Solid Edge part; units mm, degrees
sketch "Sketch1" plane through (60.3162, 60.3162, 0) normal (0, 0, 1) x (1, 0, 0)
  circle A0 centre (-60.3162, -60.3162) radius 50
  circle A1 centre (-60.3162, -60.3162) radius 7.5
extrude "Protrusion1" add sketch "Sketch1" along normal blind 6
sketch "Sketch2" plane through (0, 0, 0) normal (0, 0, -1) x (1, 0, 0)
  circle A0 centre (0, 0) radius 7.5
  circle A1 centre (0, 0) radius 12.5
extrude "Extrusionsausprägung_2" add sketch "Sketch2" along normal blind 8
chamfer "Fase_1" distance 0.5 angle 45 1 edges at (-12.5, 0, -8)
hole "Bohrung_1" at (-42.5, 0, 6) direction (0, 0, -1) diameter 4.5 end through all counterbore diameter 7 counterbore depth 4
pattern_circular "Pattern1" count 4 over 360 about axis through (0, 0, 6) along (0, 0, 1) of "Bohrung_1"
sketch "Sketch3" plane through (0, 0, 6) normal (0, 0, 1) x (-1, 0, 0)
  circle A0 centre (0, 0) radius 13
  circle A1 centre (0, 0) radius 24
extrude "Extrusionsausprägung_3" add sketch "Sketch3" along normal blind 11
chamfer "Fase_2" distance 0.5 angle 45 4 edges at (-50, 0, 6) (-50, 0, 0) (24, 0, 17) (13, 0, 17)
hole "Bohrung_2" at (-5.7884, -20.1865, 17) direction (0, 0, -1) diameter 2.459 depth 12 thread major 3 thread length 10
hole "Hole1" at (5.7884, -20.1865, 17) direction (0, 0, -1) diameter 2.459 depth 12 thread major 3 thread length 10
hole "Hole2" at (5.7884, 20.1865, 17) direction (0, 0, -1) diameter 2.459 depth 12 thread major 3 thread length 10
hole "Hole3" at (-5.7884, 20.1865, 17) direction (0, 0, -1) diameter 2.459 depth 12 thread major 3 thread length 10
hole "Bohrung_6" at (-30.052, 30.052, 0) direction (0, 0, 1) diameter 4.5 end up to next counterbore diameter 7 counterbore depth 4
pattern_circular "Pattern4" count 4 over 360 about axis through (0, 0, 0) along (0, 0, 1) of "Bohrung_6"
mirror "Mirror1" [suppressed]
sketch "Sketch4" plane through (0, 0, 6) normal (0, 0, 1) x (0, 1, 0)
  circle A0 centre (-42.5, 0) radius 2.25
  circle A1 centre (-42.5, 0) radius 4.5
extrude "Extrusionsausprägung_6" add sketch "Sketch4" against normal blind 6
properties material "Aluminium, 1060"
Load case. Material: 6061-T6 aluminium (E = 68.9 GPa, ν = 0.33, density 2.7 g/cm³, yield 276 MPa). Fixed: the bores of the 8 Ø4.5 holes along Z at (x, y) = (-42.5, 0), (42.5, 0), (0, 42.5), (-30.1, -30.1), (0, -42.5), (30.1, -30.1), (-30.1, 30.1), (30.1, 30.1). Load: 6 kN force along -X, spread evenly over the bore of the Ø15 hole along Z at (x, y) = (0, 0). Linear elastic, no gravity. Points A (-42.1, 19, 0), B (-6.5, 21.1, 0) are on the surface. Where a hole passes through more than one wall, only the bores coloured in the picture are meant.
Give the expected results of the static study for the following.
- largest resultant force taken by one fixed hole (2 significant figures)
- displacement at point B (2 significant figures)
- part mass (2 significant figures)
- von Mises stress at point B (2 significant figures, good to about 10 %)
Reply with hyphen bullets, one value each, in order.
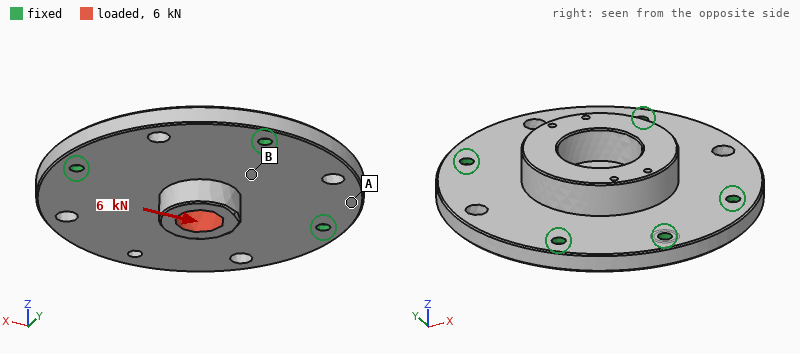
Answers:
- 920 N
- 4.9 µm
- 160 g
- 12 MPa
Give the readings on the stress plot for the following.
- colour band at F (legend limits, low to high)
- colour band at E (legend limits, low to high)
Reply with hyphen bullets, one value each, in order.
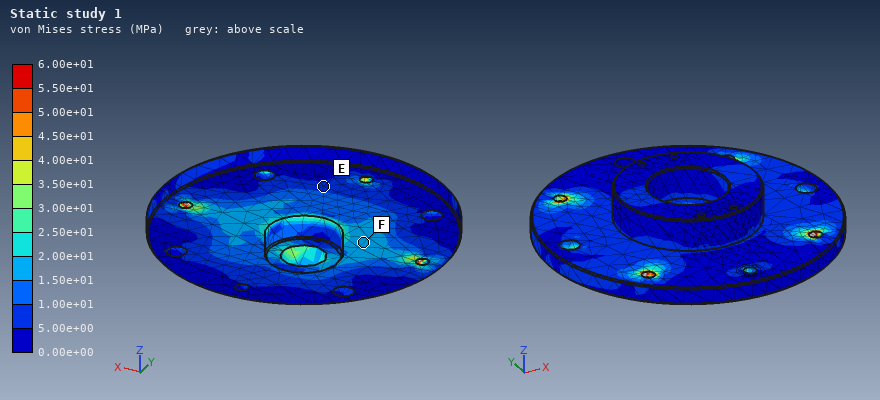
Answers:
- 1.50e+01 to 2.00e+01 MPa
- 5.00e+00 to 1.00e+01 MPa
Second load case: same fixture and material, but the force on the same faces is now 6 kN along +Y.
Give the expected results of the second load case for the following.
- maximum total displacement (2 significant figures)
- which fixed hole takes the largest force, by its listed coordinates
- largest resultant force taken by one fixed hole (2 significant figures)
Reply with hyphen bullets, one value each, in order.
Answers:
- 17 µm
- (0, -42.5)
- 1.4 kN
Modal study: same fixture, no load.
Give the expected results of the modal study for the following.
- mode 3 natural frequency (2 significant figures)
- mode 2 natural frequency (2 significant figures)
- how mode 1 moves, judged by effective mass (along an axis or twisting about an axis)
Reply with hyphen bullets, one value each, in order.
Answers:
- 10 kHz
- 10 kHz
- along Z
